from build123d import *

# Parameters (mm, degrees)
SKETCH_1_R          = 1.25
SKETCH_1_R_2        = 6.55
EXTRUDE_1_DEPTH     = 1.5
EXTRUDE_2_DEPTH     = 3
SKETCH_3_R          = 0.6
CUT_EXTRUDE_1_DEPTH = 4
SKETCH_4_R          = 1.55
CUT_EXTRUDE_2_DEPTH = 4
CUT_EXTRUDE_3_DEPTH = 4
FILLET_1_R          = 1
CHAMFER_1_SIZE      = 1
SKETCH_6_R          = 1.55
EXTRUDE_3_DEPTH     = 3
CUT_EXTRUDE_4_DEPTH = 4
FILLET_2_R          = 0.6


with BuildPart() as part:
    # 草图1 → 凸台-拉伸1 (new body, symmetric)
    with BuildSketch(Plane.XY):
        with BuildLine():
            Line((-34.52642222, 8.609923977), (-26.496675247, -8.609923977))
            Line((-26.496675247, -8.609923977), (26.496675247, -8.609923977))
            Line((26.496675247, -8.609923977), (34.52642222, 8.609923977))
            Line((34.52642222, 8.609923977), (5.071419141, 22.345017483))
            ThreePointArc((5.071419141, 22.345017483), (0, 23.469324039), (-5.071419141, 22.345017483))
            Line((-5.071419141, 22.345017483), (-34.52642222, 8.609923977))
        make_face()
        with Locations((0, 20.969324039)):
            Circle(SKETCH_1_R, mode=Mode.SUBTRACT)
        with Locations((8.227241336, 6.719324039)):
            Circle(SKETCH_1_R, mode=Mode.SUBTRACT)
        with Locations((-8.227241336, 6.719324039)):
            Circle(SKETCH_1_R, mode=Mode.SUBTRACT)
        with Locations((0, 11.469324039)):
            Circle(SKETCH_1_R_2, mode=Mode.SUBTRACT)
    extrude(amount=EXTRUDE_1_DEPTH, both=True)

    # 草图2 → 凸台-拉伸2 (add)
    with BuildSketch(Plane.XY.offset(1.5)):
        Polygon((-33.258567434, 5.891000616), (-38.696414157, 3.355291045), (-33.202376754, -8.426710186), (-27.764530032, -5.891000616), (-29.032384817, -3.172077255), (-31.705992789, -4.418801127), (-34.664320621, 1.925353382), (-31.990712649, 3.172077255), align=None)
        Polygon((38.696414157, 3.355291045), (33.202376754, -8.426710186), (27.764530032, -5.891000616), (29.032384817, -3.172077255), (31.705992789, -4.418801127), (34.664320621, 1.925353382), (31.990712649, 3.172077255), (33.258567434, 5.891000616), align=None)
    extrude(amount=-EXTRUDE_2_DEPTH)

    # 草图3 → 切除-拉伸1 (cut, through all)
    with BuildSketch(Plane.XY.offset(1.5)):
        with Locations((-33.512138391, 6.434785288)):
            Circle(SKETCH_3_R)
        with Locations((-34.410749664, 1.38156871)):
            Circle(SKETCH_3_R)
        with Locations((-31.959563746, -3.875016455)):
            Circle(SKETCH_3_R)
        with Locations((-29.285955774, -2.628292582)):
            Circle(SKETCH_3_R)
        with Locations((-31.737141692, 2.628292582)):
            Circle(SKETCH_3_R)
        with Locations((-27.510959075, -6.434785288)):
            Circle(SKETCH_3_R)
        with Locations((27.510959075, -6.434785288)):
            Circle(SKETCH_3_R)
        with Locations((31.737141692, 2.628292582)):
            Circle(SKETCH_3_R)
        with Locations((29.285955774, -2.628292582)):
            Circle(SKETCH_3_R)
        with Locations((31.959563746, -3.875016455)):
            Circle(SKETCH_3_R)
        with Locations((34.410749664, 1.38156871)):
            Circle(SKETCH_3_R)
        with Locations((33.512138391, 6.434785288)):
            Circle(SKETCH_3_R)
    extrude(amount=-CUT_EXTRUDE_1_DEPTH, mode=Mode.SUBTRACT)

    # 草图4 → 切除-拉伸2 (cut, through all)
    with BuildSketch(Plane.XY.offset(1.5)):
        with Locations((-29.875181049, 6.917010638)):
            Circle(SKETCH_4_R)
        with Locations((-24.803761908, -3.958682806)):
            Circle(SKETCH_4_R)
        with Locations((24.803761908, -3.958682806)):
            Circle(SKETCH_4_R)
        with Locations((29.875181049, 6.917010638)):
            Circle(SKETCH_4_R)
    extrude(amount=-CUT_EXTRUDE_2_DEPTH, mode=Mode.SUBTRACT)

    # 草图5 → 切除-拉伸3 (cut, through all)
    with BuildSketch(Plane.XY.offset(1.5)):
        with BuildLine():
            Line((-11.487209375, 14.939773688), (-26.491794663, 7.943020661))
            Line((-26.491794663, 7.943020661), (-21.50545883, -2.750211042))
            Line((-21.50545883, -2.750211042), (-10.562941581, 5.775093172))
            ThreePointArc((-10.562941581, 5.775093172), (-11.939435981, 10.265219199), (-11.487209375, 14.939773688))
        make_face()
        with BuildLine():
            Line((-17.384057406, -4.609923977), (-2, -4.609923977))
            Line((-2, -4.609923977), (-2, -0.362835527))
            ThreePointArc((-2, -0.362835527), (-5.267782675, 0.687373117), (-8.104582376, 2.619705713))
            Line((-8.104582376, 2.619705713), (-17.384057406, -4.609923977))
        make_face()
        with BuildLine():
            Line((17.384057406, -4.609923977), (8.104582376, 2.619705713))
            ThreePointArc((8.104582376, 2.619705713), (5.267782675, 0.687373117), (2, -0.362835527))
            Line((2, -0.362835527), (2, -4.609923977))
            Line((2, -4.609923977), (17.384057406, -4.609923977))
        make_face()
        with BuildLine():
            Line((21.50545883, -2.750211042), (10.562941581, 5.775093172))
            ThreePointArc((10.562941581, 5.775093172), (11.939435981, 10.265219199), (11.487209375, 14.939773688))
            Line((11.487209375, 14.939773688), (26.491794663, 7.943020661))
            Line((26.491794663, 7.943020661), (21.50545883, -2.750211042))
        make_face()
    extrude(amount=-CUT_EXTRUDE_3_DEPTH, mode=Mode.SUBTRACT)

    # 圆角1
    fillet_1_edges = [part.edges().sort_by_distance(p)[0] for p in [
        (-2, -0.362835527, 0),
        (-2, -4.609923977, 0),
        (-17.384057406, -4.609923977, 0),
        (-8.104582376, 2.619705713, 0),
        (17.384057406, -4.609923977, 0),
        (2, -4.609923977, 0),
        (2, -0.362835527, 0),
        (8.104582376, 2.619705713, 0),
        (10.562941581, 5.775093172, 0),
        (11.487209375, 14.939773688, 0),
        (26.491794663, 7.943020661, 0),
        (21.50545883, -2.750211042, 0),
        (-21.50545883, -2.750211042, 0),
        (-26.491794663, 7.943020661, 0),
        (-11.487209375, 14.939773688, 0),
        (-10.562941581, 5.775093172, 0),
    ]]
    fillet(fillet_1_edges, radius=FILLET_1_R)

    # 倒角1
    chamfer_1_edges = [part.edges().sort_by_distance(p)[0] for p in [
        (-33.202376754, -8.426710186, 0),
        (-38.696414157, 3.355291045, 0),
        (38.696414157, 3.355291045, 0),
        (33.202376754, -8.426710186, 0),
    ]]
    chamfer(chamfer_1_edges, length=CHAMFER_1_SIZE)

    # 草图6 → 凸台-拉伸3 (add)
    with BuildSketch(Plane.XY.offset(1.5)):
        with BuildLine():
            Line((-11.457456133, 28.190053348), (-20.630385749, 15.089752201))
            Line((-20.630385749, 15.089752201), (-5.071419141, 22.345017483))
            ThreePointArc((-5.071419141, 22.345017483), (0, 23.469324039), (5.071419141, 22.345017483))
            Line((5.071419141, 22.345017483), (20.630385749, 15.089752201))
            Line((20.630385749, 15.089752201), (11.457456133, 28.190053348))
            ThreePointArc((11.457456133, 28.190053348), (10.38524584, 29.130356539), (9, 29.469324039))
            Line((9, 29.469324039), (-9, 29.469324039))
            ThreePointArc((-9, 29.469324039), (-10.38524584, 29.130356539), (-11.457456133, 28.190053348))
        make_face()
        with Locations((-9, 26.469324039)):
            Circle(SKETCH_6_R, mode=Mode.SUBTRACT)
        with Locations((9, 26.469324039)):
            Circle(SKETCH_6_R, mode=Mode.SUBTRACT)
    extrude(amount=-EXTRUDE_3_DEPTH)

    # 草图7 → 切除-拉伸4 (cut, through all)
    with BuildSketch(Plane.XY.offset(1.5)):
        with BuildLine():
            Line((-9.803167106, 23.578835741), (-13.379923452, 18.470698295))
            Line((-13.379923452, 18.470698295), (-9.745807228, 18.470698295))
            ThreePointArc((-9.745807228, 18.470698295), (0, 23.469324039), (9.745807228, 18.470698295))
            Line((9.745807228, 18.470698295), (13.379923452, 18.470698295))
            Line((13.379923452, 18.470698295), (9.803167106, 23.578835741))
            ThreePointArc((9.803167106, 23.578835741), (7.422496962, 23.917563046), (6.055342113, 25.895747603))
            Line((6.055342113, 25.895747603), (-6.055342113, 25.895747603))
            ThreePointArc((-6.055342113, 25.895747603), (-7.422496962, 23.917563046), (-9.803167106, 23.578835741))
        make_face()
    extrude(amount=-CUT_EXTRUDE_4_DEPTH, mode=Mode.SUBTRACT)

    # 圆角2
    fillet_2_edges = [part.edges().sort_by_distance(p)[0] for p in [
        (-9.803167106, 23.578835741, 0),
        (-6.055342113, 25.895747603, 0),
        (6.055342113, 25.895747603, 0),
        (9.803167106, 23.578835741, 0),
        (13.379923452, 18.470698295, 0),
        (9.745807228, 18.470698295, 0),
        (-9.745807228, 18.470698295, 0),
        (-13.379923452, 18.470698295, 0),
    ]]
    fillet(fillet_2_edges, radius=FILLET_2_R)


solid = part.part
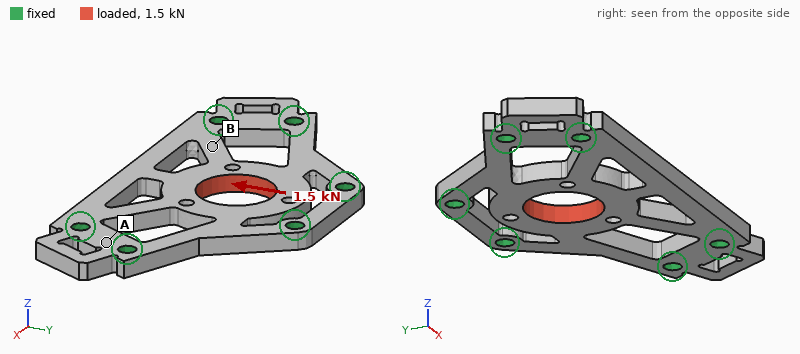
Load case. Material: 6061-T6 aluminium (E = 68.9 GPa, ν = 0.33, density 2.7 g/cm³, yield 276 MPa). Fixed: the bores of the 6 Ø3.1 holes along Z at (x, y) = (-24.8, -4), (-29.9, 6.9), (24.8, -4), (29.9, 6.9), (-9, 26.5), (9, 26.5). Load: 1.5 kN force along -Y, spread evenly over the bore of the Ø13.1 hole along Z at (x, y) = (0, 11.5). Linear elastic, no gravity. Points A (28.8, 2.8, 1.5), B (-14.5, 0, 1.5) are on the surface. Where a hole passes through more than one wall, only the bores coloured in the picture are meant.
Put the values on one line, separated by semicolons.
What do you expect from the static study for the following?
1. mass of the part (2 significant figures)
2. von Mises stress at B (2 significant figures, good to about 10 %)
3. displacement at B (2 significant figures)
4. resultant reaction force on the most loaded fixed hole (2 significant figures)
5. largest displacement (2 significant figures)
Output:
10 g; 37 MPa; 13 µm; 390 N; 28 µm
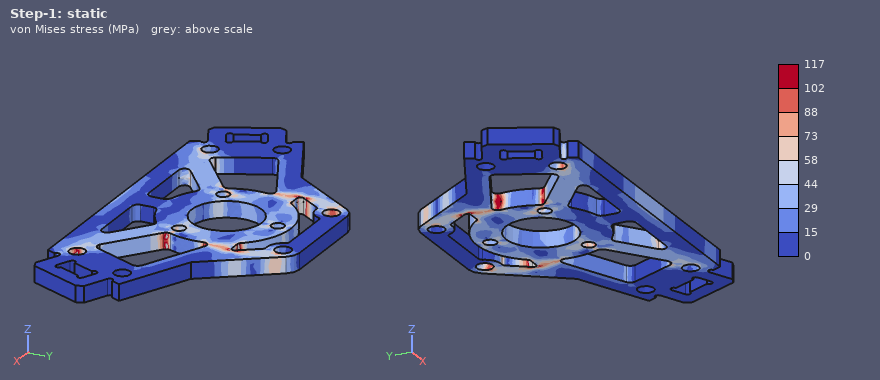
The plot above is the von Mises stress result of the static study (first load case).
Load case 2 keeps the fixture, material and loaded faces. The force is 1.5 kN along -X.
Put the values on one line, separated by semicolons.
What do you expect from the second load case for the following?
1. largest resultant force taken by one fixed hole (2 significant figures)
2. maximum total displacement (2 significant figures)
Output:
400 N; 15 µm
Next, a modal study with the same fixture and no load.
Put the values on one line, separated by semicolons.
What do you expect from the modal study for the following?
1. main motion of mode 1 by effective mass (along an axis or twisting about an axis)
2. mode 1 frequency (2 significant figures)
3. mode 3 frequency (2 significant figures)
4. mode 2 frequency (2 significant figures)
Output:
along Z; 6100 Hz; 14 kHz; 9200 Hz
